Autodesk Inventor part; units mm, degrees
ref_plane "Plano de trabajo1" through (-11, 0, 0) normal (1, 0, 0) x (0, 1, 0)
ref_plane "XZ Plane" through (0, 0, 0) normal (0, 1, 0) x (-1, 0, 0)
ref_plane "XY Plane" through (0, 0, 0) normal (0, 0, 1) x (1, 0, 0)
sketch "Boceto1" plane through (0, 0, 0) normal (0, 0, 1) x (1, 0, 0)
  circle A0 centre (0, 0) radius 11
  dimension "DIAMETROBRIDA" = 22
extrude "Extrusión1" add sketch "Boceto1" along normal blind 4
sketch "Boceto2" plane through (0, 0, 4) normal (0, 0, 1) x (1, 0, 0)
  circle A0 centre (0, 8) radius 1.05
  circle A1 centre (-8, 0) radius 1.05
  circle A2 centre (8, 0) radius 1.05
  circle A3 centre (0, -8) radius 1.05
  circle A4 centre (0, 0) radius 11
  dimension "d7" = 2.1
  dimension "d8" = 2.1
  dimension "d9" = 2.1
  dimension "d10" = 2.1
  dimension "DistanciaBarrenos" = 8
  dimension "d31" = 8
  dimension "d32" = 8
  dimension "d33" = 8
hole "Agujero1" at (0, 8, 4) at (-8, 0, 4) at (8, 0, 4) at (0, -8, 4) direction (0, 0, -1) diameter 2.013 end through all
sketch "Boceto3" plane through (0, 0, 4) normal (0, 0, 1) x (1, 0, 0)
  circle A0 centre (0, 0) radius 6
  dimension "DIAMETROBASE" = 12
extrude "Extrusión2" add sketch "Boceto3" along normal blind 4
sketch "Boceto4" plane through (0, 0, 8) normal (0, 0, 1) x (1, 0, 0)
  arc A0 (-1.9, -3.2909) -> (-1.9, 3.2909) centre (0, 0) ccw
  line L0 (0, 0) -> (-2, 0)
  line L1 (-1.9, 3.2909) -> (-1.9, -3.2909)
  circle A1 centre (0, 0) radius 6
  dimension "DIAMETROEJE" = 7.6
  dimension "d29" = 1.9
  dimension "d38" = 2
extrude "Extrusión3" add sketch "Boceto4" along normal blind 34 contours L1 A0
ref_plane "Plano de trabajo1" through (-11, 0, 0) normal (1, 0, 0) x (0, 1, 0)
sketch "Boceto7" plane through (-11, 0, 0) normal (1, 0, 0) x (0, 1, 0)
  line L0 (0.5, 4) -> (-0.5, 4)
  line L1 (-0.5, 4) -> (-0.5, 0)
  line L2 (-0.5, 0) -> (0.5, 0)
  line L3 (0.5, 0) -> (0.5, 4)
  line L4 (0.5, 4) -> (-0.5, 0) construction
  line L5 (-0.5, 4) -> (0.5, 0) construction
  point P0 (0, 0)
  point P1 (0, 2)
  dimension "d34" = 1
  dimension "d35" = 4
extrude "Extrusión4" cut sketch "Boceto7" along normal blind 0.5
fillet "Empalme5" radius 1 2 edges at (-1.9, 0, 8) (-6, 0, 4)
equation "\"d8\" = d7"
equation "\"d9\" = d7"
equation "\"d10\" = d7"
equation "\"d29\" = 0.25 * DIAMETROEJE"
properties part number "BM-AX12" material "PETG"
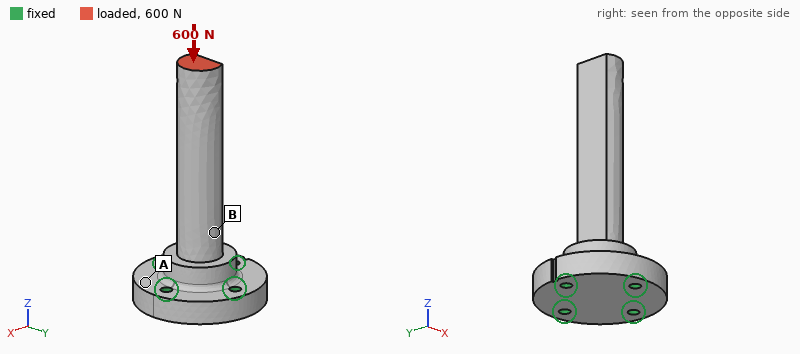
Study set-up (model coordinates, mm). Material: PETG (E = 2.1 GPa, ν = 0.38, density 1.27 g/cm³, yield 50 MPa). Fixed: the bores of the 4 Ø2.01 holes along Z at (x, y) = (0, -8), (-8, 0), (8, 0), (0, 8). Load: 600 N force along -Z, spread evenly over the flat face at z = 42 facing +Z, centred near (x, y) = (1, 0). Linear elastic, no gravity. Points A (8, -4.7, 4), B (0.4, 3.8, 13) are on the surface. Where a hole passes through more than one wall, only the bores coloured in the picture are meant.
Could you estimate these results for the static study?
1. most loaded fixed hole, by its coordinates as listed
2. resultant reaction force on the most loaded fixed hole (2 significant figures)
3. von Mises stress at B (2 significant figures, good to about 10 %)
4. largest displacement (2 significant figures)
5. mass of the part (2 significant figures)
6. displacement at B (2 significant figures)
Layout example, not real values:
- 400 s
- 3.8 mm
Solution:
- (8, 0)
- 180 N
- 16 MPa
- 0.32 mm
- 4.0 g
- 0.084 mm
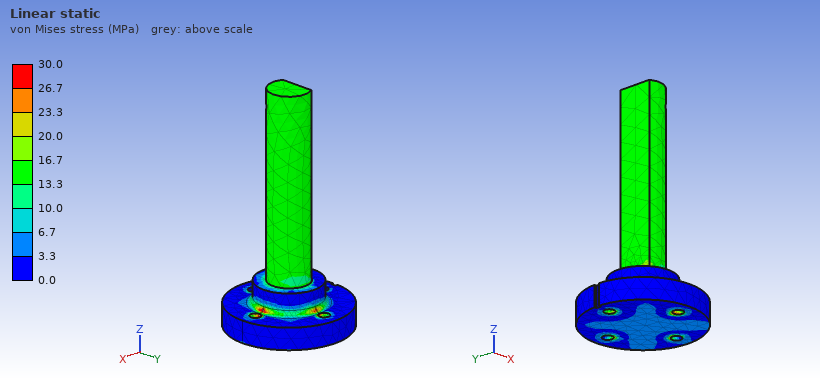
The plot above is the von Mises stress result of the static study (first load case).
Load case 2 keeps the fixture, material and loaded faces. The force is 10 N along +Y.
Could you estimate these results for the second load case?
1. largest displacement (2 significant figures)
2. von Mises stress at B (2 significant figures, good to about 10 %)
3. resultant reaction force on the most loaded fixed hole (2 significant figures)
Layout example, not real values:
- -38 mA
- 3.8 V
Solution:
- 0.54 mm
- 7.6 MPa
- 25 N
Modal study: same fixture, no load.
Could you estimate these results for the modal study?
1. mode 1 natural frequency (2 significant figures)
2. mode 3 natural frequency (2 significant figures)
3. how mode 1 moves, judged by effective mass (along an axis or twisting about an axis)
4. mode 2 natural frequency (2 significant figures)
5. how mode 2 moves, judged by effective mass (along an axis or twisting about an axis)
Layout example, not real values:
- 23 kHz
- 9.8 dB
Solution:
- 850 Hz
- 4800 Hz
- along X
- 1100 Hz
- along Y
